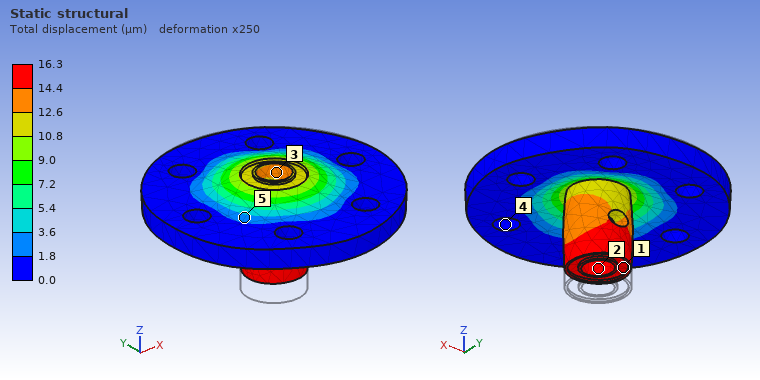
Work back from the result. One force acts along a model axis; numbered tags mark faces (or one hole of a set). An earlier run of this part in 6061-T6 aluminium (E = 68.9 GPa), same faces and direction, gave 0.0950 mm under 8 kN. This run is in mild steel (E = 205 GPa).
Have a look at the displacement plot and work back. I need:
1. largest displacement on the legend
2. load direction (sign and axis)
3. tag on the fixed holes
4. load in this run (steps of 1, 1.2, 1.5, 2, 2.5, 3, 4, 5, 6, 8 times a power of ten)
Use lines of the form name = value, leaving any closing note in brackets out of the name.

largest displacement on the legend = 16.3 µm
load direction = +Z
tag on the fixed holes = 4
load in this run = 4 kN
